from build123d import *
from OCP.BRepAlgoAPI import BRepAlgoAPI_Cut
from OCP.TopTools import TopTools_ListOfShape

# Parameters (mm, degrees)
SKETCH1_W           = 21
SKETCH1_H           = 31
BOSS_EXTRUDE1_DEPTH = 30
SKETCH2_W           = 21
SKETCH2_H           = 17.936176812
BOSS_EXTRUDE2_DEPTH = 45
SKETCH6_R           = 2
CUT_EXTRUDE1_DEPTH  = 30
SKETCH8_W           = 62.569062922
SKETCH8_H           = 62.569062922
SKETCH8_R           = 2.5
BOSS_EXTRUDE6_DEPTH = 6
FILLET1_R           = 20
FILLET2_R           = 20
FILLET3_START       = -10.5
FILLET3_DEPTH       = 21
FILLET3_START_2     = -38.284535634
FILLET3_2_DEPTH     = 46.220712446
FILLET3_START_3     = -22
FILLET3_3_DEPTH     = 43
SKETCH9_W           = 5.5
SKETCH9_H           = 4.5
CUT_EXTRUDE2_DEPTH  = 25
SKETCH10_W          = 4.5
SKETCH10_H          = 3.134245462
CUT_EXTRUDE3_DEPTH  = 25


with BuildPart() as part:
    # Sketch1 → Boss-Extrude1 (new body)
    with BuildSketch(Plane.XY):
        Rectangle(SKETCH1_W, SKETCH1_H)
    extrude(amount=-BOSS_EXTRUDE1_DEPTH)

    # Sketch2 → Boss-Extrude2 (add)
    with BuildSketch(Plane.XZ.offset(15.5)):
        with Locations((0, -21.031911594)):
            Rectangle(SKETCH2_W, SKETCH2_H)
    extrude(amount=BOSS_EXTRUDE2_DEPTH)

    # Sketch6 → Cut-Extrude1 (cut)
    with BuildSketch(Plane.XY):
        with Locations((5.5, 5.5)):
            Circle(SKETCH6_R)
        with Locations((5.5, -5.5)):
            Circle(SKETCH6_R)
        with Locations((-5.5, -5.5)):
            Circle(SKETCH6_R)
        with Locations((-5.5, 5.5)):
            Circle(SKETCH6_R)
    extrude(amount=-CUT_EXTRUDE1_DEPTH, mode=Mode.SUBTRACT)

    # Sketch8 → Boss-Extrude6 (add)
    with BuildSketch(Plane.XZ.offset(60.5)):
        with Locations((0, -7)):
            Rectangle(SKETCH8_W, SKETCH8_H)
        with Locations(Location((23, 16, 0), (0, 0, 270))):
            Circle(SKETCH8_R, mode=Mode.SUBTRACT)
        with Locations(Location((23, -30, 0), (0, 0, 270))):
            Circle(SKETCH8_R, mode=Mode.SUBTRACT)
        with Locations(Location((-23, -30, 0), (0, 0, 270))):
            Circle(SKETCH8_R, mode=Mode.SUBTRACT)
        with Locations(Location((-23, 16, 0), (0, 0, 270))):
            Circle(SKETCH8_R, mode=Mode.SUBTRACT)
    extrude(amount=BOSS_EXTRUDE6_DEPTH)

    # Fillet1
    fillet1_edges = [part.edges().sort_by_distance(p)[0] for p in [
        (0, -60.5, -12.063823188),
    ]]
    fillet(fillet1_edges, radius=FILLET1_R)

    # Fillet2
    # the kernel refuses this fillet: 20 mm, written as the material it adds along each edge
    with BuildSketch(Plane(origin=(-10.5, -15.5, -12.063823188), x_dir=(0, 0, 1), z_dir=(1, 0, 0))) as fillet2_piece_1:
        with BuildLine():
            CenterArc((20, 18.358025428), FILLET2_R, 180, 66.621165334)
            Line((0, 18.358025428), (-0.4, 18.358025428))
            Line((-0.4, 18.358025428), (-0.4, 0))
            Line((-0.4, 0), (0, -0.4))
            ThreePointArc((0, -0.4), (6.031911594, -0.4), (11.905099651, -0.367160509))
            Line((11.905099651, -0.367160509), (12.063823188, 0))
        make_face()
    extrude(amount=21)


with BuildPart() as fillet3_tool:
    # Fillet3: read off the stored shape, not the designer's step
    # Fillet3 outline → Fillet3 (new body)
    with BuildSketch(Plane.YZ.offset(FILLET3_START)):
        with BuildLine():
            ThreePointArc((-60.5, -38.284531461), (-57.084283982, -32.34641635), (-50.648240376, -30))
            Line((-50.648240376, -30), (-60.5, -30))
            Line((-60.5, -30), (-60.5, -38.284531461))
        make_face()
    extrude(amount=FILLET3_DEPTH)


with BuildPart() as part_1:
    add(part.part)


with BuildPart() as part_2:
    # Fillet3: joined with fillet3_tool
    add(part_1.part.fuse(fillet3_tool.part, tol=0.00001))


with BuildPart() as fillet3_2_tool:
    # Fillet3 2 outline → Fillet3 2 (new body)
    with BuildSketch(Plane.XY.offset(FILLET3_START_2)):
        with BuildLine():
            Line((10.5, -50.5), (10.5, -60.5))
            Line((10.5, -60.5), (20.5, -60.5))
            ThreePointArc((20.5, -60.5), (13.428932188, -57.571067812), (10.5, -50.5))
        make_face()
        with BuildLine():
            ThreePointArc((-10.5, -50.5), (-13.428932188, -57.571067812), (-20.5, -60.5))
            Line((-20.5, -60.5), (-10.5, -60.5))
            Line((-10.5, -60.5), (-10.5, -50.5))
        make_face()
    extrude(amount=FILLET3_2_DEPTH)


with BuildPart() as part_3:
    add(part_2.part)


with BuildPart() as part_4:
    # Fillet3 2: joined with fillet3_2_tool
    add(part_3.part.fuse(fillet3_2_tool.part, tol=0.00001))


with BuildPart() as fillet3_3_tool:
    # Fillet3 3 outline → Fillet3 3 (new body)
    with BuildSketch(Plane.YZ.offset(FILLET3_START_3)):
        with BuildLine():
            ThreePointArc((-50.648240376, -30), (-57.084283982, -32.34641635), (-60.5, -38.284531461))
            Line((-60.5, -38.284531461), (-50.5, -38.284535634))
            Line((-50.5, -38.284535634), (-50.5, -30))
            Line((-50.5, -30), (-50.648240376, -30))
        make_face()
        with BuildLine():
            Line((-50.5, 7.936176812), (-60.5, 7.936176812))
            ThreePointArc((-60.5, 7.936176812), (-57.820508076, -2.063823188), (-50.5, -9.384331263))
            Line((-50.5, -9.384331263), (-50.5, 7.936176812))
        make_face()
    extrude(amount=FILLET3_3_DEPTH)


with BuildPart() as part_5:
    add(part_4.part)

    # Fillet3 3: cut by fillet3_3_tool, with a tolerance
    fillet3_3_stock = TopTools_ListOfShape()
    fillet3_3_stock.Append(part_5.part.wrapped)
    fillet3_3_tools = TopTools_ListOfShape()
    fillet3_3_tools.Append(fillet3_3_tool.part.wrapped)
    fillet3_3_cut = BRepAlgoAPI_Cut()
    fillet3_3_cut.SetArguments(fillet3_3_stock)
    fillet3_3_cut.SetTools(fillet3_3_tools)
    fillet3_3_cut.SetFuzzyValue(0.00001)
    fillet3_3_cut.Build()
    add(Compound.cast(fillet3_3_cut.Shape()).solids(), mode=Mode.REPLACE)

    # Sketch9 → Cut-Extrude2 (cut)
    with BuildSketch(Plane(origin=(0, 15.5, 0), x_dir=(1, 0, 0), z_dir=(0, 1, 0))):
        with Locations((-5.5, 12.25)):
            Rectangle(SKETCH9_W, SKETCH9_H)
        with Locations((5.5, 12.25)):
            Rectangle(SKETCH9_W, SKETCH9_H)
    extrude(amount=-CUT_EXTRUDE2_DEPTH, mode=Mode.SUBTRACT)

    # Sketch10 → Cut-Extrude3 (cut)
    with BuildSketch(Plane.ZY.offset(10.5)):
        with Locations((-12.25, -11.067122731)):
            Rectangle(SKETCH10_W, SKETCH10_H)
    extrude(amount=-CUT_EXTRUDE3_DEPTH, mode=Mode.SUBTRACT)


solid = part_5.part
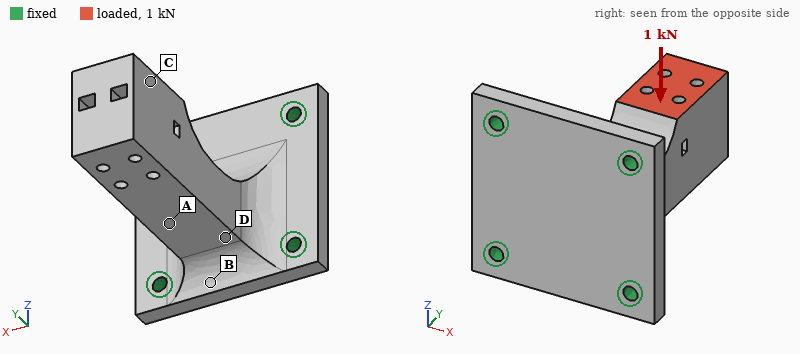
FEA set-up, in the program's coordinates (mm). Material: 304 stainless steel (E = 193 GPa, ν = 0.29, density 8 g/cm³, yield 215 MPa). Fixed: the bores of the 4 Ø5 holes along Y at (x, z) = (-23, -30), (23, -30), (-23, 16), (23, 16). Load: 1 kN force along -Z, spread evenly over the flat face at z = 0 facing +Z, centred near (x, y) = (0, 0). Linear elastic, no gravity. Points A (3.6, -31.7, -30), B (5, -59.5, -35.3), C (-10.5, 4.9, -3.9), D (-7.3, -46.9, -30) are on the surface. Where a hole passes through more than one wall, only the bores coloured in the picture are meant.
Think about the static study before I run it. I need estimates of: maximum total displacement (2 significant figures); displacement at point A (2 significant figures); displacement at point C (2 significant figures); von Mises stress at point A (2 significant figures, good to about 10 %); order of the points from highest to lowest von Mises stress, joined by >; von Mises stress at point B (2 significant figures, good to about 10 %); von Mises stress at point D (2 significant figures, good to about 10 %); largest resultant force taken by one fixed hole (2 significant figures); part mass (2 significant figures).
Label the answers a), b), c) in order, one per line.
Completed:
a) 74 µm
b) 21 µm
c) 62 µm
d) 27 MPa
e) D > A > B > C
f) 14 MPa
g) 38 MPa
h) 830 N
i) 490 g
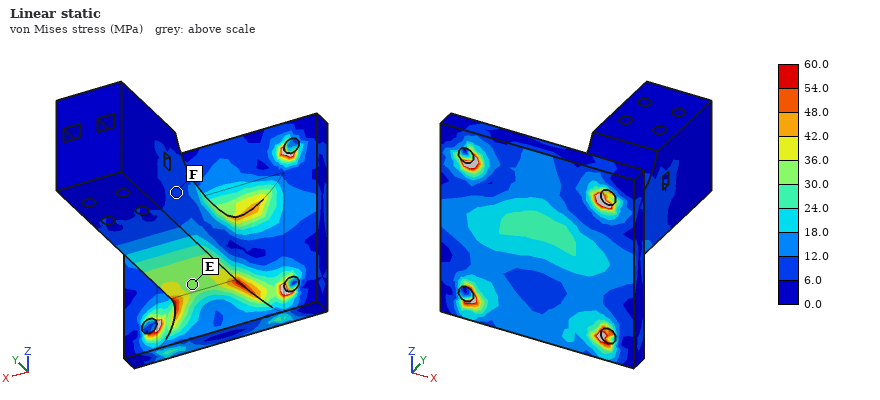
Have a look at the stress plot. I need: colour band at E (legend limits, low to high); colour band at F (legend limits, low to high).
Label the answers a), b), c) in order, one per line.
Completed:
a) 30.0 to 36.0 MPa
b) 6.0 to 12.0 MPa
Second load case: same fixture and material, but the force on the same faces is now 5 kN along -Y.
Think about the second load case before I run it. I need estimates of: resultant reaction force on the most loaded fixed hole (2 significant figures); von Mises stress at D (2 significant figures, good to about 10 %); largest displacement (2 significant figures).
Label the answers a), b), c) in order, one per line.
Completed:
a) 1.8 kN
b) 69 MPa
c) 0.17 mm
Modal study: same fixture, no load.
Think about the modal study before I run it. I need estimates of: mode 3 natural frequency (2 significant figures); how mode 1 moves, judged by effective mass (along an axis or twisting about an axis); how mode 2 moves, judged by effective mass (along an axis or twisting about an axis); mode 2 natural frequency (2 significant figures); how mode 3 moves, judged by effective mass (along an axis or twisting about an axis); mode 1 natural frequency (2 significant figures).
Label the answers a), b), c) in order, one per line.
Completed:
a) 6400 Hz
b) along Z
c) along X
d) 2000 Hz
e) along Y
f) 1700 Hz
